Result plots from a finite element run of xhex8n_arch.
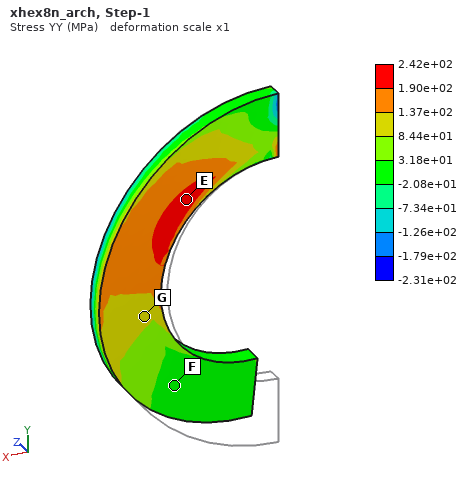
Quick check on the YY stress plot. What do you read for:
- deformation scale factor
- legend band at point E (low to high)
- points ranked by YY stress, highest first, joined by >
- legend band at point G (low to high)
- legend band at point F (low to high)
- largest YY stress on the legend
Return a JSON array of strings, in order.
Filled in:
["1", "1.90e+02 to 2.42e+02 MPa", "E > G > F", "8.44e+01 to 1.37e+02 MPa", "-2.08e+01 to 3.18e+01 MPa", "2.42e+02 MPa"]
